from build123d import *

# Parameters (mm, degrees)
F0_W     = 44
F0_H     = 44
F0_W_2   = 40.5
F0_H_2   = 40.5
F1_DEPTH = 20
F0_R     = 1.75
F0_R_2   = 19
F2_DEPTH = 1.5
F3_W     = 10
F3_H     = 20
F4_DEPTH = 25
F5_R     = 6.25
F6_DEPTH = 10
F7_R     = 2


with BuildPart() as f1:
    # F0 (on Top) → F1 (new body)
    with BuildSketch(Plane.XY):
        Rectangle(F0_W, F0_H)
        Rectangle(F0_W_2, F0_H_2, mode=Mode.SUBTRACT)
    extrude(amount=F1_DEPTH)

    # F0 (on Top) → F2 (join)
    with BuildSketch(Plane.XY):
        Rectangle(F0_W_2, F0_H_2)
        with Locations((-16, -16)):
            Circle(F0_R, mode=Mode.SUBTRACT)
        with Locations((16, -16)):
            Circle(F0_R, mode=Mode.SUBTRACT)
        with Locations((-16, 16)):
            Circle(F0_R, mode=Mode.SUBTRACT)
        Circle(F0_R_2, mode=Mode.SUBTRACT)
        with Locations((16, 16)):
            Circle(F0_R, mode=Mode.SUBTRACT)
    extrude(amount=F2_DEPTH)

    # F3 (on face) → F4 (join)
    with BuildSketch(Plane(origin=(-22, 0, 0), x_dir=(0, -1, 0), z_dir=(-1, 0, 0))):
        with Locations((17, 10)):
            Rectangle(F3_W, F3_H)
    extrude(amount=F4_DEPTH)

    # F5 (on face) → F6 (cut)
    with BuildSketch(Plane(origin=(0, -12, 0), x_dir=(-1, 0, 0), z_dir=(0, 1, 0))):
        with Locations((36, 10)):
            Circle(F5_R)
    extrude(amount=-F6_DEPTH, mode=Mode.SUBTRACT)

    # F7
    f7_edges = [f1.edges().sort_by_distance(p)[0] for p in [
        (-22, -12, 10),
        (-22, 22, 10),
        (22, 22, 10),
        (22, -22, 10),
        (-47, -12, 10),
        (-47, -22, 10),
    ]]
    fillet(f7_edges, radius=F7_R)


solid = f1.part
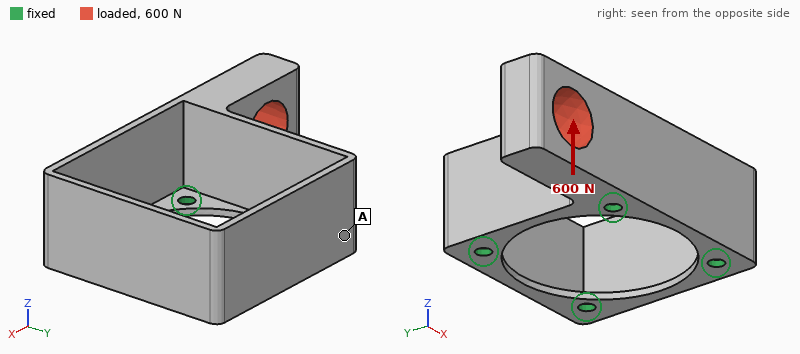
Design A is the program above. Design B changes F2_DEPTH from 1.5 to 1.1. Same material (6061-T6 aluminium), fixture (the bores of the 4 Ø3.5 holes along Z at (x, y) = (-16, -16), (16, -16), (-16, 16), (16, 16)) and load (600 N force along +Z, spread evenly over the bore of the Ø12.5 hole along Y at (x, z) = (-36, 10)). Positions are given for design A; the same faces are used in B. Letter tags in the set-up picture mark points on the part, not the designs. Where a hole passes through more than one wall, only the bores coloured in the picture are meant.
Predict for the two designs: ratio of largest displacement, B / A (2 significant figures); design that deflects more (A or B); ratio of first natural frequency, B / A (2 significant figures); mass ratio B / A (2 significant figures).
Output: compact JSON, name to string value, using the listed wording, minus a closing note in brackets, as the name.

{"ratio of largest displacement, B / A": "1.3", "design that deflects more": "B", "ratio of first natural frequency, B / A": "0.89", "mass ratio B / A": "0.98"}
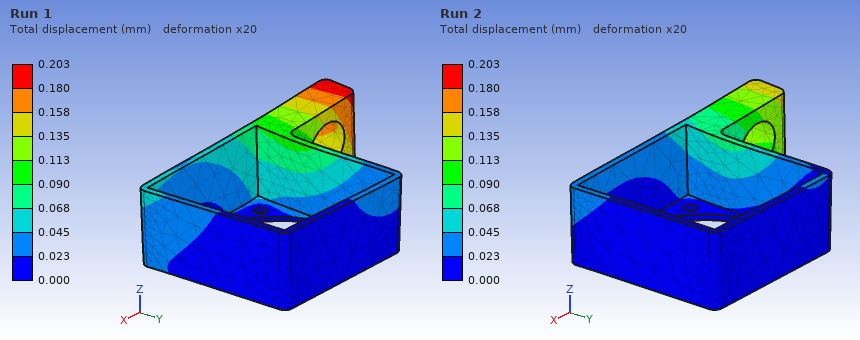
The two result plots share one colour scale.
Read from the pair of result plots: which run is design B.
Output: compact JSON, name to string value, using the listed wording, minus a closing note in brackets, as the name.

{"which run is design B": "Run 1"}
